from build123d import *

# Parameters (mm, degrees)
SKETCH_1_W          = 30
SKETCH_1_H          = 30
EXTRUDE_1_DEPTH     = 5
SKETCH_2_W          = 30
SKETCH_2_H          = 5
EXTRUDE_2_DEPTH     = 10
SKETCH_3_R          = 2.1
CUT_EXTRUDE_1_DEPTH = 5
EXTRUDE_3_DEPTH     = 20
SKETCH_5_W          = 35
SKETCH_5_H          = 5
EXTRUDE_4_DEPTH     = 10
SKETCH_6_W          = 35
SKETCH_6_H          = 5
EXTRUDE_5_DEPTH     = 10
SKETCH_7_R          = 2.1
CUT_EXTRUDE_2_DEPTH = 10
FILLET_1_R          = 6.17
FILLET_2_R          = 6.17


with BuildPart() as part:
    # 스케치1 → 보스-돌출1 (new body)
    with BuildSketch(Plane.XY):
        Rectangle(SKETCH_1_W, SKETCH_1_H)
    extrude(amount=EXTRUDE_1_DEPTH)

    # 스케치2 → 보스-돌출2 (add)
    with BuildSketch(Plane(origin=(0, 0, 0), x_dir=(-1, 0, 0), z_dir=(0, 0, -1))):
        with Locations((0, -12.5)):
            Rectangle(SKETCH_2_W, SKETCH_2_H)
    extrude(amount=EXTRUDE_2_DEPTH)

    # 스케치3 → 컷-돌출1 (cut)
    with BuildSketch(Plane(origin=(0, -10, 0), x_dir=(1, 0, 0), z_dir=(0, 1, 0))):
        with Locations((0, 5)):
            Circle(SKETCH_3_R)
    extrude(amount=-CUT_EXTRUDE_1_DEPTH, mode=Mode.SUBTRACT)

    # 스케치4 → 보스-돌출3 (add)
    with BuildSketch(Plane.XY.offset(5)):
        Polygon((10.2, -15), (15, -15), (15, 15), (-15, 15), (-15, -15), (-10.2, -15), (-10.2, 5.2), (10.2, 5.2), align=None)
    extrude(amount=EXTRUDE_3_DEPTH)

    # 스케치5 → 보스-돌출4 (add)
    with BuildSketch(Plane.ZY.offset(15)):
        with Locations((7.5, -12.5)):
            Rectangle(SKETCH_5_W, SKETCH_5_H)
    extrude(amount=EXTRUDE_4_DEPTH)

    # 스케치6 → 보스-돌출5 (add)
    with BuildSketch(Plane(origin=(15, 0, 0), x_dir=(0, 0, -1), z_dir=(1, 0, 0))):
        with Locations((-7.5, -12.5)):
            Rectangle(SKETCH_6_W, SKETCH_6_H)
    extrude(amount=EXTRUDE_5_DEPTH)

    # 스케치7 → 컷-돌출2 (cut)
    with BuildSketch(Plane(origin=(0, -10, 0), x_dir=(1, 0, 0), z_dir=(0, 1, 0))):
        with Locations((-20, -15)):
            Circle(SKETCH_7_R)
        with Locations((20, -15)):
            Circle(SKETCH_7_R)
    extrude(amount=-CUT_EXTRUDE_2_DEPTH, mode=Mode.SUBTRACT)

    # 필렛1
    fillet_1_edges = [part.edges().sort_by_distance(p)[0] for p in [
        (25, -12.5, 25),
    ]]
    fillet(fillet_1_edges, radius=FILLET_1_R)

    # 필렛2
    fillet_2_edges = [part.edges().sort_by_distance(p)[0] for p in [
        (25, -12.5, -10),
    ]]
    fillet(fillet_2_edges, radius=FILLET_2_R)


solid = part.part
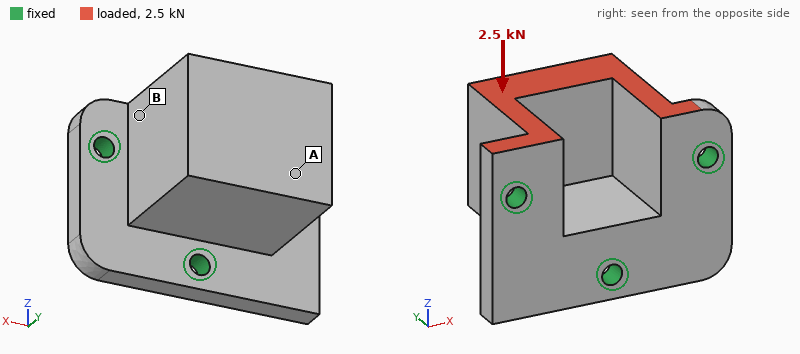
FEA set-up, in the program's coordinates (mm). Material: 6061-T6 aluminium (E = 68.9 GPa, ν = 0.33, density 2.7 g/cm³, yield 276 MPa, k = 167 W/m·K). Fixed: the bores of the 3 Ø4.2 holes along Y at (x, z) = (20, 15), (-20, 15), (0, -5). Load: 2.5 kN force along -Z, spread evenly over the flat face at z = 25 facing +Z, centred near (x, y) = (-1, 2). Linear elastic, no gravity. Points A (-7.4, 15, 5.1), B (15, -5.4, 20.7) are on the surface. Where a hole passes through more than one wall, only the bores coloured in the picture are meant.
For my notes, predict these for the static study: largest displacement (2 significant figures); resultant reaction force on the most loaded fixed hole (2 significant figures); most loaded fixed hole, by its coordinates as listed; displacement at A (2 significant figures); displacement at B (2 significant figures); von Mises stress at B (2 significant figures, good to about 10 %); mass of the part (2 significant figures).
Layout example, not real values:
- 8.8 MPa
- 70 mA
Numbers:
- 46 µm
- 1.8 kN
- (0, -5)
- 40 µm
- 19 µm
- 29 MPa
- 51 g
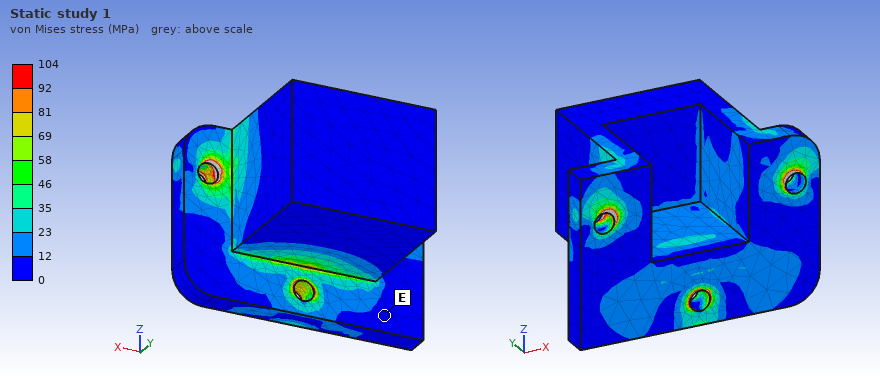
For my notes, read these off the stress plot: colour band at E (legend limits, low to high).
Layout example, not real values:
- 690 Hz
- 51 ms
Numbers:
- 0 to 12 MPa
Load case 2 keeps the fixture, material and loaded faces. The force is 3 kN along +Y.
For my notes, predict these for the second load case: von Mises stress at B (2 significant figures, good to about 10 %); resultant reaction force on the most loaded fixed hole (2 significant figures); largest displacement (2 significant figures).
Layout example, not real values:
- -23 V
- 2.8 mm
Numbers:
- 55 MPa
- 2.1 kN
- 64 µm
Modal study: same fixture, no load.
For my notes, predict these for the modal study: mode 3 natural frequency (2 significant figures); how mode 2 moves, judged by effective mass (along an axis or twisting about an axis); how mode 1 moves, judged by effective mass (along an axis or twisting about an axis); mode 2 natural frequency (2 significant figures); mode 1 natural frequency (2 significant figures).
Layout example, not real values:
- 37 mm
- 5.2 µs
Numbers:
- 13 kHz
- along X
- along Z
- 7300 Hz
- 6600 Hz
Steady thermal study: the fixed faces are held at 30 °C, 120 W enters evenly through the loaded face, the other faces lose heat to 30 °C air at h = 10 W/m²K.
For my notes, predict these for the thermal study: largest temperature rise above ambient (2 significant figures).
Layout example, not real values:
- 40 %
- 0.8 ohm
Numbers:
- 57 K
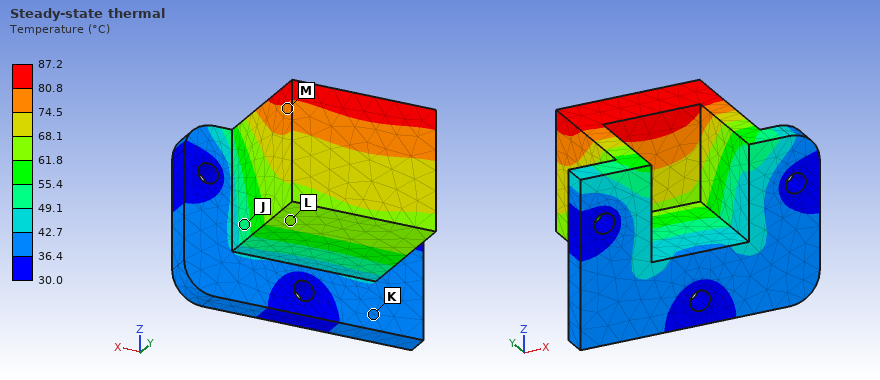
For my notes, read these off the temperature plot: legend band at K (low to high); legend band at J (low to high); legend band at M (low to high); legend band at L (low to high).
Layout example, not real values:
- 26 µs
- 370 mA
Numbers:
- 36.4 to 42.7 °C
- 49.1 to 55.4 °C
- 74.5 to 80.8 °C
- 61.8 to 68.1 °C
